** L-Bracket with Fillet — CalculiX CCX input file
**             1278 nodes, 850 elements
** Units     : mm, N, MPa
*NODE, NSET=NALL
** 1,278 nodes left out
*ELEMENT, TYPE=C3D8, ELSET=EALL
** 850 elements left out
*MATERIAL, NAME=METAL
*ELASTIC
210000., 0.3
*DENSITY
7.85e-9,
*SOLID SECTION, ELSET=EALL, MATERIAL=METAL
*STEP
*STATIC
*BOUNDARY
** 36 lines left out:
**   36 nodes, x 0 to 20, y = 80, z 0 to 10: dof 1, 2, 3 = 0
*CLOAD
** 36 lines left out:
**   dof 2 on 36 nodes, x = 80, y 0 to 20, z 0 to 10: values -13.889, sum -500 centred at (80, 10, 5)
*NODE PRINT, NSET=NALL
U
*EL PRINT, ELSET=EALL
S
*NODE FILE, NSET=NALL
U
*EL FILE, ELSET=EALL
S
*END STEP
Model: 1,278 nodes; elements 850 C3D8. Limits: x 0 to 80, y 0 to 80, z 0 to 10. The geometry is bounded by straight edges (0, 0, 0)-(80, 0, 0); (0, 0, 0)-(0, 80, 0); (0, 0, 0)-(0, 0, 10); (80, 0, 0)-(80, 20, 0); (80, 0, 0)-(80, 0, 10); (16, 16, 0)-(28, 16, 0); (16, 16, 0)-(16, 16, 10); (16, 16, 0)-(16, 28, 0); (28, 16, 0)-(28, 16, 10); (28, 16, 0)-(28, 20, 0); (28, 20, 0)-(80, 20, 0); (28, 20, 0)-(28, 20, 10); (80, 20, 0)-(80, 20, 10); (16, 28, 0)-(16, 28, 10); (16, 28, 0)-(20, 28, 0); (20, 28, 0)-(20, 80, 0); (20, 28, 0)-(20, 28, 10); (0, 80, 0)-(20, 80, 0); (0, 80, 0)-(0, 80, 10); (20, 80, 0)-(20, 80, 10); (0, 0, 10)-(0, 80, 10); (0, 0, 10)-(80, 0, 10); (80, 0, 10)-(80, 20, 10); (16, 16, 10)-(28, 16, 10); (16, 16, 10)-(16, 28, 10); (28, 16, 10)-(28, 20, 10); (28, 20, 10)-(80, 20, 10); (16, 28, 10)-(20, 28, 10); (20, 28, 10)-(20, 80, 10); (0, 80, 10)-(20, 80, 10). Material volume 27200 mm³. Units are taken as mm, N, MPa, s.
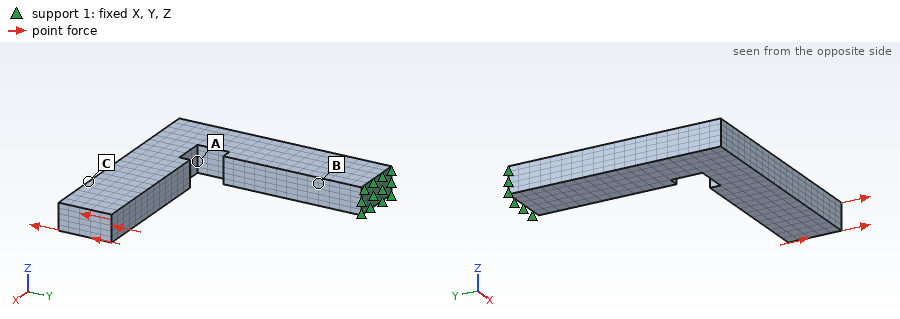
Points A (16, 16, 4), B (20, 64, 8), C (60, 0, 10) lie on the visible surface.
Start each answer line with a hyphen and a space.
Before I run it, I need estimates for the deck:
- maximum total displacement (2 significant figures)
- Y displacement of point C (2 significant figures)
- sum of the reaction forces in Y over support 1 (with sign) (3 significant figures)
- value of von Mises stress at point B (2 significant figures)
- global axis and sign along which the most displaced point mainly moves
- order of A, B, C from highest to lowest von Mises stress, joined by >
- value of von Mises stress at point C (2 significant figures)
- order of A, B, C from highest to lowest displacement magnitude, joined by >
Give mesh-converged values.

- 0.25 mm
- -0.16 mm
- 500 N
- 55 MPa
- -Y
- A > B > C
- 15 MPa
- C > A > B
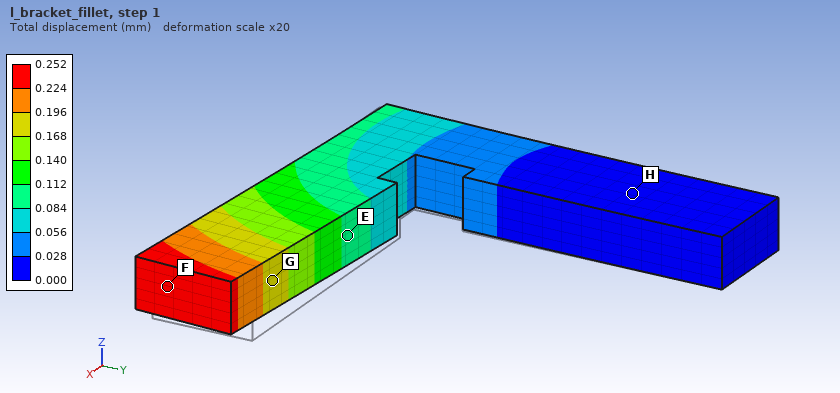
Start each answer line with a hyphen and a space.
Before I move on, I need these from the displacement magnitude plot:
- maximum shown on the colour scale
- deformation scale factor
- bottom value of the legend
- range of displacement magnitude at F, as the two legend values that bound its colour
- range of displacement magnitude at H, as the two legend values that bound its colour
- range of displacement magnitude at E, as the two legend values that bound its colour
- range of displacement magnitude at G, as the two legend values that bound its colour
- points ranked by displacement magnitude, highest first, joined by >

- 0.252 mm
- 20
- 0.000 mm
- 0.224 to 0.252 mm
- 0.000 to 0.028 mm
- 0.084 to 0.112 mm
- 0.168 to 0.196 mm
- F > G > E > H
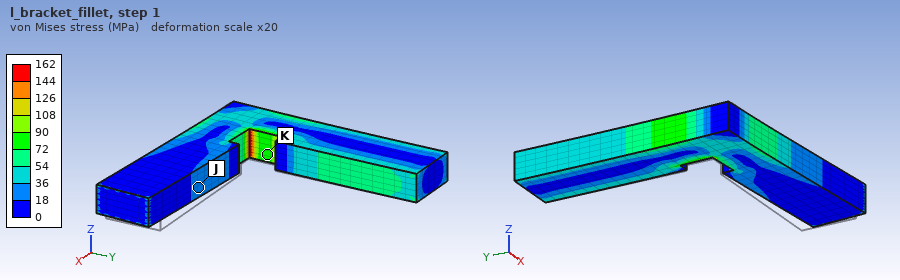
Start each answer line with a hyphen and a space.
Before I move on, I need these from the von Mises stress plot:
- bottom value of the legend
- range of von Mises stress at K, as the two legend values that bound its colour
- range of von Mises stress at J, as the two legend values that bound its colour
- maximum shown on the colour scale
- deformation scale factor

- 0 MPa
- 72 to 90 MPa
- 18 to 36 MPa
- 162 MPa
- 20
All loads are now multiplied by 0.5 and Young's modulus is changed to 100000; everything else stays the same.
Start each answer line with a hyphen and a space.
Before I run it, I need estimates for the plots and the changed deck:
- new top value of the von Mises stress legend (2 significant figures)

- 81 MPa
